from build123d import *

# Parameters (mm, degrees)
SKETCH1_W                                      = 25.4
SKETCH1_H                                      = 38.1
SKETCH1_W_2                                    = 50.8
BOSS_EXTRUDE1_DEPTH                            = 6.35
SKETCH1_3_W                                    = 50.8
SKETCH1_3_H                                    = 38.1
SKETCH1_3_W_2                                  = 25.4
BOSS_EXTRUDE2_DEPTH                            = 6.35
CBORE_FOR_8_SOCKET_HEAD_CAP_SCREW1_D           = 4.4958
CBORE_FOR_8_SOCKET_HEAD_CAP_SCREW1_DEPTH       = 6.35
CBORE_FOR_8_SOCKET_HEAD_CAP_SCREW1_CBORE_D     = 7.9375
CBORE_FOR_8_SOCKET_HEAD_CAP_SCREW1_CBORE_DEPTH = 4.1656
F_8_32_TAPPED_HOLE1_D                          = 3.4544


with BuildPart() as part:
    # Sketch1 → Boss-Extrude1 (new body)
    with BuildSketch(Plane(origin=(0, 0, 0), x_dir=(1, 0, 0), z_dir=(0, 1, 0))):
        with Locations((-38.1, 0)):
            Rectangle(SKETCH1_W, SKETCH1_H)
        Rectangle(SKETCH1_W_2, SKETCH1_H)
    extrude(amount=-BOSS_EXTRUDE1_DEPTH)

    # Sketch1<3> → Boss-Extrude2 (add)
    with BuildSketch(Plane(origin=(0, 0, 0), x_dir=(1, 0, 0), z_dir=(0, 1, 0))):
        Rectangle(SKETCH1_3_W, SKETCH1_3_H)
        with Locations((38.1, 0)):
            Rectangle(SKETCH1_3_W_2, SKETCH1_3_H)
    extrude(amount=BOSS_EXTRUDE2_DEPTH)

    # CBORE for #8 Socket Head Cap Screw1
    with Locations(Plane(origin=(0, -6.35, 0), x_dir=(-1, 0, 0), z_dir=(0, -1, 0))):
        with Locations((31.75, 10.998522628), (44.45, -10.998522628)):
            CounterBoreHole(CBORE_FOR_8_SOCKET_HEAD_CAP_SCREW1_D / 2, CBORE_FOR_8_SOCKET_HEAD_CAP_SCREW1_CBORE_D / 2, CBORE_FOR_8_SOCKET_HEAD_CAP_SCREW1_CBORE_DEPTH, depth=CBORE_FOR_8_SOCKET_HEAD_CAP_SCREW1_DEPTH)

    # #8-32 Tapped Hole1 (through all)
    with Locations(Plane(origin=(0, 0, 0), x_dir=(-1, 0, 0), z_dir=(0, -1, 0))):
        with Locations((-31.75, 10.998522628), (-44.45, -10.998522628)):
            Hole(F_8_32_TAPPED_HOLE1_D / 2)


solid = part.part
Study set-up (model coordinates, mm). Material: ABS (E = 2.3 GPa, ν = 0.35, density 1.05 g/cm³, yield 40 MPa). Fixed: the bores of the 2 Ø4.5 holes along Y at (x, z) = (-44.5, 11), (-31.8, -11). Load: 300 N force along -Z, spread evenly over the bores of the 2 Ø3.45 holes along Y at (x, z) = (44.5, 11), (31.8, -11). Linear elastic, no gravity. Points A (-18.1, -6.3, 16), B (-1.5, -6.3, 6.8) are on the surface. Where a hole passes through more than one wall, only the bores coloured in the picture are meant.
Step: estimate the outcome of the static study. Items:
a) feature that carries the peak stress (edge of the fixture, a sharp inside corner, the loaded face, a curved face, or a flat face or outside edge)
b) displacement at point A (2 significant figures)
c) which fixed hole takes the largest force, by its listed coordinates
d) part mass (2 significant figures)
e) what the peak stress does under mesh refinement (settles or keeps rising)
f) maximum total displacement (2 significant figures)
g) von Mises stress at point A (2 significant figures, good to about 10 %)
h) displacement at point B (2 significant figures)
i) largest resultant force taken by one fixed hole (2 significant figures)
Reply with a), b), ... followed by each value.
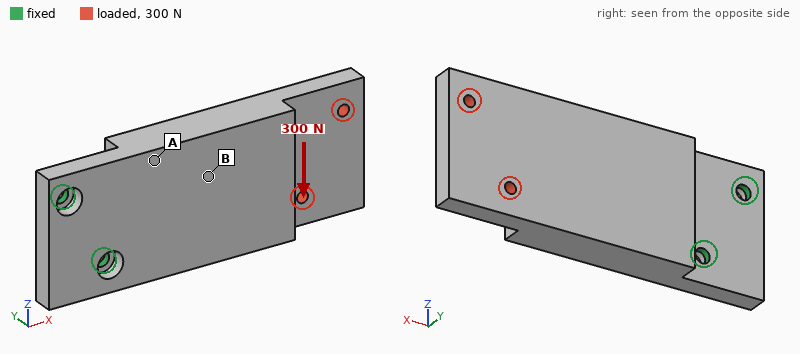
a) edge of the fixture
b) 0.30 mm
c) (-31.8, -11)
d) 38 g
e) keeps rising
f) 1.2 mm
g) 6.8 MPa
h) 0.36 mm
i) 910 N
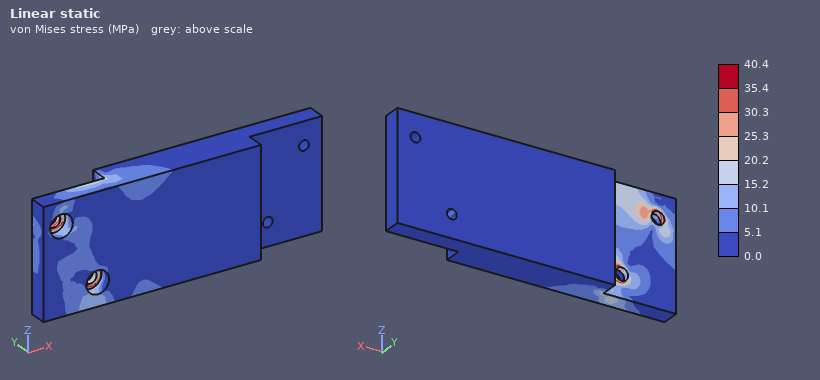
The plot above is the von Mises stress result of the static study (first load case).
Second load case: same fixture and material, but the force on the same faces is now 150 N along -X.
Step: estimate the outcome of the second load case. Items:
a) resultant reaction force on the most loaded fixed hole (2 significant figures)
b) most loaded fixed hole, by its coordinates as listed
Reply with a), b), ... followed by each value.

a) 83 N
b) (-31.8, -11)
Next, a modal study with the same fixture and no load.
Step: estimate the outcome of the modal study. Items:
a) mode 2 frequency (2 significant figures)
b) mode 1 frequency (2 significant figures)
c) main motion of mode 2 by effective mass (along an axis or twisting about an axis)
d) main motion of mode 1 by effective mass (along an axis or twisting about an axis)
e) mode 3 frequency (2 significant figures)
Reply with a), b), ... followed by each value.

a) 760 Hz
b) 160 Hz
c) along Z
d) along Y
e) 1100 Hz
